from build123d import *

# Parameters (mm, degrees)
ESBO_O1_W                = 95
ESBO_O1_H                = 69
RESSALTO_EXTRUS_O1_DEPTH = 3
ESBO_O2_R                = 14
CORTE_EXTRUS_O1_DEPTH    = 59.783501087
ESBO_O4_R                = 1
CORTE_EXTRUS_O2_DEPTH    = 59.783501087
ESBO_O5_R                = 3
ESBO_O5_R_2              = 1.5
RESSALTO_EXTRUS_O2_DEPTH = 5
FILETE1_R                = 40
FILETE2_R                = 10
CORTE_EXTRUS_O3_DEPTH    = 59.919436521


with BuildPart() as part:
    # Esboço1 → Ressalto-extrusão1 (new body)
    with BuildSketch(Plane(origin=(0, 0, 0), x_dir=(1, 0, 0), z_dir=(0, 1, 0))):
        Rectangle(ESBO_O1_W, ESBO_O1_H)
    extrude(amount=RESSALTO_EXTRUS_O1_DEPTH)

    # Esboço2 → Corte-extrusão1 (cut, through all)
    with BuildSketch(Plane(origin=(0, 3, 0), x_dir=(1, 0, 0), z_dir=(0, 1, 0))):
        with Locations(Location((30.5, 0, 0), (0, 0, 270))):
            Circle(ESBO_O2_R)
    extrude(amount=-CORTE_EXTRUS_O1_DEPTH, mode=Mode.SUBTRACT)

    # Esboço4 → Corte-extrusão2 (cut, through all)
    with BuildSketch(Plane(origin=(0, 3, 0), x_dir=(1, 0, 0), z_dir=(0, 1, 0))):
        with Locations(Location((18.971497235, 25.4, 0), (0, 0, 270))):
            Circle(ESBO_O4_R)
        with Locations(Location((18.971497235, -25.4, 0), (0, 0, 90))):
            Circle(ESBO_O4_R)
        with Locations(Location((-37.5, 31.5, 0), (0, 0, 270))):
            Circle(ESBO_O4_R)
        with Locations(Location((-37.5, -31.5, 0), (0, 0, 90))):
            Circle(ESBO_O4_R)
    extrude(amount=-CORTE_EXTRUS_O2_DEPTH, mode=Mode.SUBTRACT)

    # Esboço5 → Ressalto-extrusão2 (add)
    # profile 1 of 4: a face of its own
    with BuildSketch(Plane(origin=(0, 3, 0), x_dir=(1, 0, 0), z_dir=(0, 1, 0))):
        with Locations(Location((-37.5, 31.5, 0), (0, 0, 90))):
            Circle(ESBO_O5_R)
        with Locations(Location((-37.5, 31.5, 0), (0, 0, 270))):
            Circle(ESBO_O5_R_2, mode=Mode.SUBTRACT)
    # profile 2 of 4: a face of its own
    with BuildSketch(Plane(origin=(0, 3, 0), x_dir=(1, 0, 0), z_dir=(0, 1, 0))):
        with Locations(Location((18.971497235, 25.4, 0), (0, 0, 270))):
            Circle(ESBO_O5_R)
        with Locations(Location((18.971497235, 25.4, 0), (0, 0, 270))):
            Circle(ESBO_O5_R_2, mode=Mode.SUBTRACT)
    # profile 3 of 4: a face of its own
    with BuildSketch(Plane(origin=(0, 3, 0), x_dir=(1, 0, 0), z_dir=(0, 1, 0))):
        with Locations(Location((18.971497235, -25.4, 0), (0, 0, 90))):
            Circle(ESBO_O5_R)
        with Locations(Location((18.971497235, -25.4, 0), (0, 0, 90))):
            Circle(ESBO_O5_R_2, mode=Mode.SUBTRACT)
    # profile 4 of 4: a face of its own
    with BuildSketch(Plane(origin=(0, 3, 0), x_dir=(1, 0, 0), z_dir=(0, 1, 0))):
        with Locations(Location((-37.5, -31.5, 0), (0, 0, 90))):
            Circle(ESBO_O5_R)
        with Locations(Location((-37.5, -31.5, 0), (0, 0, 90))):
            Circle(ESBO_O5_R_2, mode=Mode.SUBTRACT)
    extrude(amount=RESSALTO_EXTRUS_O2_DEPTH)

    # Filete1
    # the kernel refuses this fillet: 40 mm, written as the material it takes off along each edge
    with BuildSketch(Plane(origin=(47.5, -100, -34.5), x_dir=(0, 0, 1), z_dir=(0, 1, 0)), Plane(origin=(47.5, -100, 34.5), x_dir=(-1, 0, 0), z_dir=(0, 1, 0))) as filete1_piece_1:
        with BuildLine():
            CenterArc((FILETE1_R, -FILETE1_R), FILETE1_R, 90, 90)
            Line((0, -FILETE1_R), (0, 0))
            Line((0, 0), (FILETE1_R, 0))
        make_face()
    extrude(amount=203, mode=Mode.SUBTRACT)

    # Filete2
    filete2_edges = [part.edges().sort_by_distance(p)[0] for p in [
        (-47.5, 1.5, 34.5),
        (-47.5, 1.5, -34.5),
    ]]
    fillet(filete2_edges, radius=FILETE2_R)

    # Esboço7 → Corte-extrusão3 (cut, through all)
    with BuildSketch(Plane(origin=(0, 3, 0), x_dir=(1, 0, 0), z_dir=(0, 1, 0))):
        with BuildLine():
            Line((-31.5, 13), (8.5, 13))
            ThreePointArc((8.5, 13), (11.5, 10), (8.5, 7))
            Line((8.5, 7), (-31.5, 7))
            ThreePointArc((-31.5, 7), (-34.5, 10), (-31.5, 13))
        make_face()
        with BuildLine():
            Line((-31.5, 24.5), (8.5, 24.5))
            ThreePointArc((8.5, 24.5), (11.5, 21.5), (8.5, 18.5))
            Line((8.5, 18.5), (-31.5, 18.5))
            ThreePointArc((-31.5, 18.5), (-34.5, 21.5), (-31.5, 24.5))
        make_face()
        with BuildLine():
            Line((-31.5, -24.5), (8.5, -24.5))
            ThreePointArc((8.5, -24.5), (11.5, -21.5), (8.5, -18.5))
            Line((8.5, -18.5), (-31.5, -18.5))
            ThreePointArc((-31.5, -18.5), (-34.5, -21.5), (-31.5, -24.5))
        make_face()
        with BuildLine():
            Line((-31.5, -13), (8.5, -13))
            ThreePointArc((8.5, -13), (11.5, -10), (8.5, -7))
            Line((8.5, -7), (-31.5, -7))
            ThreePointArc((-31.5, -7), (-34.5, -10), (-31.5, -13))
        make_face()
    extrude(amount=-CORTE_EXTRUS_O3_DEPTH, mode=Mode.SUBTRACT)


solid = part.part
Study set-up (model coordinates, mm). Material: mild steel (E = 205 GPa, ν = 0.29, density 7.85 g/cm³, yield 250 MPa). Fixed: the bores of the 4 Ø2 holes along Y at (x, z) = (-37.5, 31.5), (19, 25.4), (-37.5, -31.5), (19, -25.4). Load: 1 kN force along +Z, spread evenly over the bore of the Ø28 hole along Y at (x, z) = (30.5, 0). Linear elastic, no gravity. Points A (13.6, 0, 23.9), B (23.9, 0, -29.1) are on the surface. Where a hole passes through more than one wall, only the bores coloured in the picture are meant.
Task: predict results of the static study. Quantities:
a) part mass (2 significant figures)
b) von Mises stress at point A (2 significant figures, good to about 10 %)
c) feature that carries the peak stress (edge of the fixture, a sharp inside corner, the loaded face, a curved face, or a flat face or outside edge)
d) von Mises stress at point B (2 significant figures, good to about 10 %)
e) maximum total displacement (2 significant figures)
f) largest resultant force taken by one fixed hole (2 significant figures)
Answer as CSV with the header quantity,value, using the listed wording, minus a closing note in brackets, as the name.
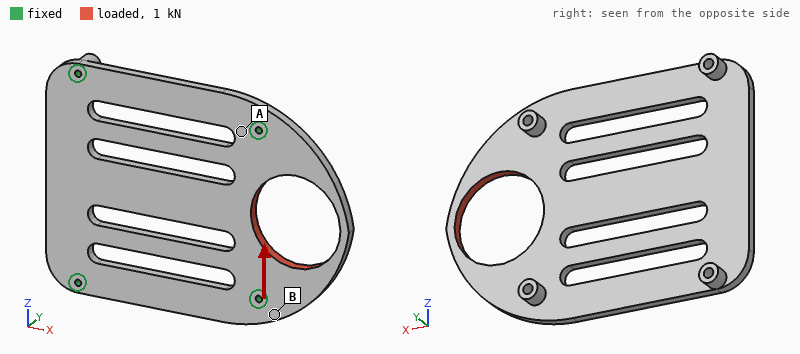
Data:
quantity,value
part mass,100 g
von Mises stress at point A,8.2 MPa
feature that carries the peak stress,edge of the fixture
von Mises stress at point B,17 MPa
maximum total displacement,11 µm
largest resultant force taken by one fixed hole,530 N
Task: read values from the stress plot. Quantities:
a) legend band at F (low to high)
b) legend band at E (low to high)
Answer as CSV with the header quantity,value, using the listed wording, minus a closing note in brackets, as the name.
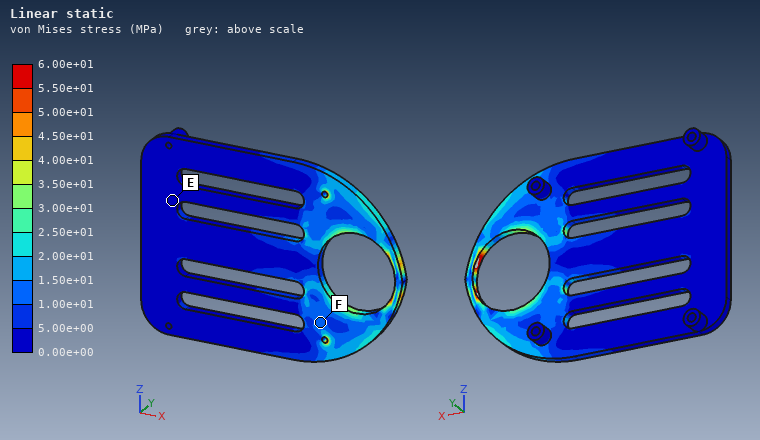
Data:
quantity,value
legend band at F,1.00e+01 to 1.50e+01 MPa
legend band at E,0.00e+00 to 5.00e+00 MPa
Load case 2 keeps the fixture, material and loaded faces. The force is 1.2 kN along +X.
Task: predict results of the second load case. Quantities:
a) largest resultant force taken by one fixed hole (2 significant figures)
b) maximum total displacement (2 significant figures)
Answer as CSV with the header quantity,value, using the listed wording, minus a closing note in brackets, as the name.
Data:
quantity,value
largest resultant force taken by one fixed hole,540 N
maximum total displacement,4.5 µm
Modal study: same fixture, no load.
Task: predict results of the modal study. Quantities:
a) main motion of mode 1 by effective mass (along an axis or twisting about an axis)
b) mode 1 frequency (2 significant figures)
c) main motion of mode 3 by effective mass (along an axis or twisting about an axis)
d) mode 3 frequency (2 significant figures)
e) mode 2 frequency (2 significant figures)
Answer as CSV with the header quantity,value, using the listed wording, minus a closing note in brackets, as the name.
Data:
quantity,value
main motion of mode 1 by effective mass,along Y
mode 1 frequency,2500 Hz
main motion of mode 3 by effective mass,twisting about Z
mode 3 frequency,4100 Hz
mode 2 frequency,3500 Hz
